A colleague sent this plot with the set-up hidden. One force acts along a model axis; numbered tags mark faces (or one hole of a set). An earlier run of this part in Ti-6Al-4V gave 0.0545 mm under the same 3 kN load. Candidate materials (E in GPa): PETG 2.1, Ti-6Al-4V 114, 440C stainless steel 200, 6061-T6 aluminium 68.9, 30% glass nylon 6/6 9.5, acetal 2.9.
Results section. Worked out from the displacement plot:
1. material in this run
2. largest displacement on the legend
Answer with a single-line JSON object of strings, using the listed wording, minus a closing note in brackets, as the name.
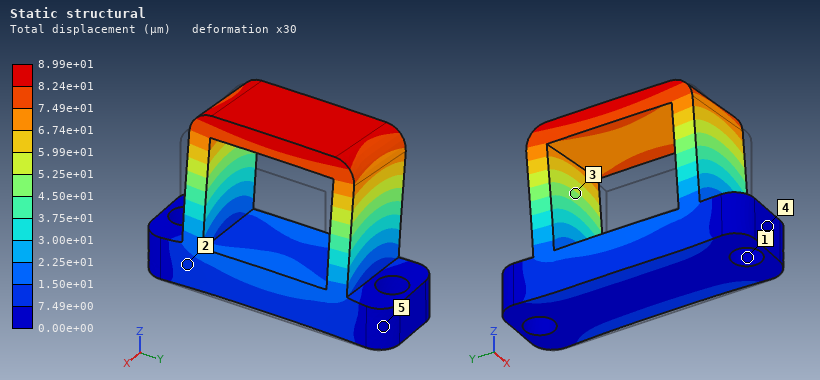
{"material in this run": "6061-T6 aluminium", "largest displacement on the legend": "8.99e+01 µm"}
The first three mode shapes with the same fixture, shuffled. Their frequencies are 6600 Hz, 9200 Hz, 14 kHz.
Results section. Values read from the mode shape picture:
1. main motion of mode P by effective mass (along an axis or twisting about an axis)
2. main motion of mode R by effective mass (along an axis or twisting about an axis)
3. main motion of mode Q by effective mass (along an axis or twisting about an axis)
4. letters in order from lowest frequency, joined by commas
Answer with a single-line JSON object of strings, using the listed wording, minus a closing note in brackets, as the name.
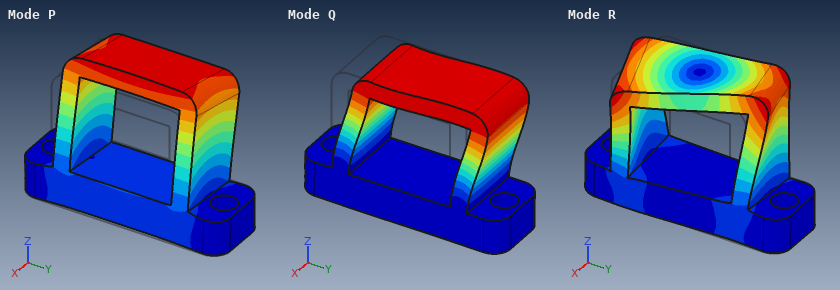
{"main motion of mode P by effective mass": "along X", "main motion of mode R by effective mass": "twisting about Z", "main motion of mode Q by effective mass": "along Y", "letters in order from lowest frequency, joined by commas": "Q, P, R"}
